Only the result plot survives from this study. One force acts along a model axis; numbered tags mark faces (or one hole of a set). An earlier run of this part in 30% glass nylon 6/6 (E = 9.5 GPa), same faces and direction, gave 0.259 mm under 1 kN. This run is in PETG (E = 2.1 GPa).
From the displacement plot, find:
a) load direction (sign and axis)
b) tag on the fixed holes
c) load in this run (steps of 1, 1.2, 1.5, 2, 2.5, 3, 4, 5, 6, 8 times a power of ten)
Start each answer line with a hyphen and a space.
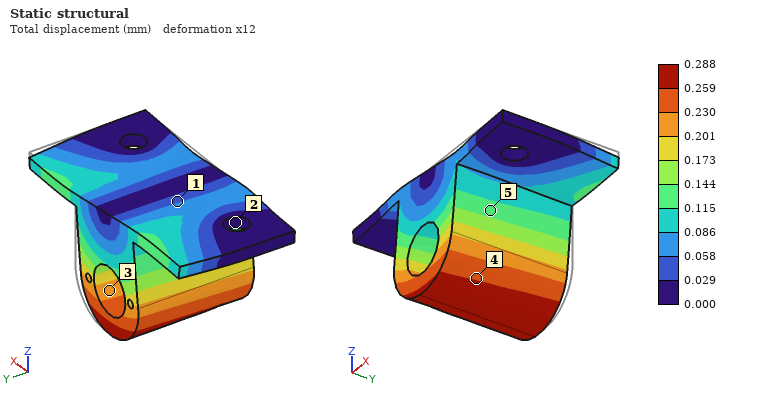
- -X
- 2
- 250 N
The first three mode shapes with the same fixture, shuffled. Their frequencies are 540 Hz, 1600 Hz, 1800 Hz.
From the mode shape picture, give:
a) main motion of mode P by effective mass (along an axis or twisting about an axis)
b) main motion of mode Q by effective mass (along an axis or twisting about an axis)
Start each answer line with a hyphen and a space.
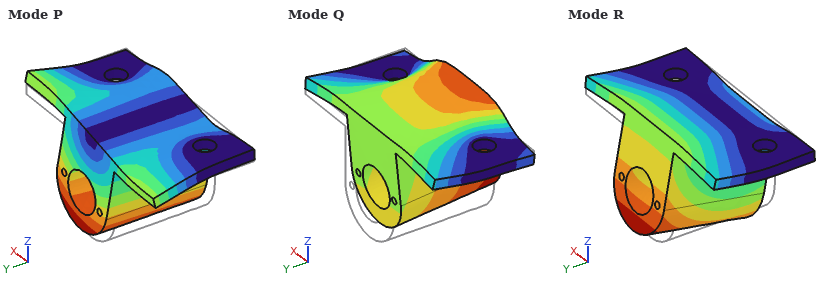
- along X
- along Z
